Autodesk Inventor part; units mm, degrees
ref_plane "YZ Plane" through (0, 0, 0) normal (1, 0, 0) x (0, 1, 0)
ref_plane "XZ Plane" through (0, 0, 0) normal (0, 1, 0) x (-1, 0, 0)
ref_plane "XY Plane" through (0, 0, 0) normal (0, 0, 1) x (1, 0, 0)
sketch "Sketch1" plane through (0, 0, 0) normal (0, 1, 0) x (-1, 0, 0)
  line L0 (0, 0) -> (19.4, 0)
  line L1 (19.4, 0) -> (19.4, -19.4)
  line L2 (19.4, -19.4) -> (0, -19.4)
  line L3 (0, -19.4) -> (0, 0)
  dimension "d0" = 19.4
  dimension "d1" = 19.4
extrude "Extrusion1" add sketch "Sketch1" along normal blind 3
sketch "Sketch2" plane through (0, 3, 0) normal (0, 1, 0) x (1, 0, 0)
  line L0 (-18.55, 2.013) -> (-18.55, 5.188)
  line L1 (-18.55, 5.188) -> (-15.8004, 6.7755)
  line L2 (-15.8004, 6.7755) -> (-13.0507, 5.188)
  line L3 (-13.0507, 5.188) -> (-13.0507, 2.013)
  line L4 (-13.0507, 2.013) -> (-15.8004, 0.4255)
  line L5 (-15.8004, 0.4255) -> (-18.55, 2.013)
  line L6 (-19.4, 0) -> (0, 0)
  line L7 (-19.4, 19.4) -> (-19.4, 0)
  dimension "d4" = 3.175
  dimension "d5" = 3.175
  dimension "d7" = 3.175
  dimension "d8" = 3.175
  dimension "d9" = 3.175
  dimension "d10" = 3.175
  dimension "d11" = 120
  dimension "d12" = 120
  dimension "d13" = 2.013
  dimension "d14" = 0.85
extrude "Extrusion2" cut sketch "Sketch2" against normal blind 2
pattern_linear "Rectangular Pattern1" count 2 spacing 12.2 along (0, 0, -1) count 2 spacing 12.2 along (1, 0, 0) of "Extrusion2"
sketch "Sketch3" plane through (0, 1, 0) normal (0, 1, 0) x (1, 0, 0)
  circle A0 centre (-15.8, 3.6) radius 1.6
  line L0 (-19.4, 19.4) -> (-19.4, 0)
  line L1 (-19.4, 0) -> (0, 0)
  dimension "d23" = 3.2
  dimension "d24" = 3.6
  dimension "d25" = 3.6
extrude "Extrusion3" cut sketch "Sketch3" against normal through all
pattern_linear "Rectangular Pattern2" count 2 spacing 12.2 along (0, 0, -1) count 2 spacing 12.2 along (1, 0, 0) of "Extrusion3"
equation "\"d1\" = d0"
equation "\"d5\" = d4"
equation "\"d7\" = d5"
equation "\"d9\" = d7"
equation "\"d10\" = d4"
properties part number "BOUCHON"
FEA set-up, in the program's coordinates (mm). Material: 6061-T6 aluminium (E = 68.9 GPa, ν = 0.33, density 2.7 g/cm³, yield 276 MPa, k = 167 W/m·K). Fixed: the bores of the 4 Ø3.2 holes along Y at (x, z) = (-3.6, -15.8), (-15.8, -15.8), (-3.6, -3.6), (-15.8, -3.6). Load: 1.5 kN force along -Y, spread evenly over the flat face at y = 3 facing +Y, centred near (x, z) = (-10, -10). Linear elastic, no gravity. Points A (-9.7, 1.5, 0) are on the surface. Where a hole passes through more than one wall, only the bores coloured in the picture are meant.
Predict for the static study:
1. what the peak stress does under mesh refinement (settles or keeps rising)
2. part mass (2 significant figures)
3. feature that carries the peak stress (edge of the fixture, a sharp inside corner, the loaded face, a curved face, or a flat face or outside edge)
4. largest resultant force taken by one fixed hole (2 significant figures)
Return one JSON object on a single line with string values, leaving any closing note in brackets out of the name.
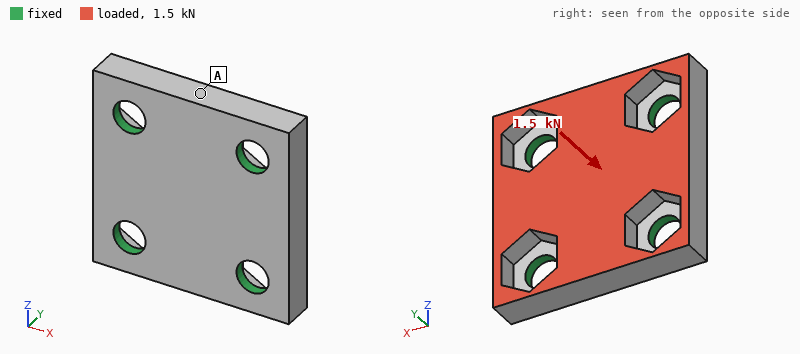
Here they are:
{"what the peak stress does under mesh refinement": "keeps rising", "part mass": "2.4 g", "feature that carries the peak stress": "edge of the fixture", "largest resultant force taken by one fixed hole": "400 N"}
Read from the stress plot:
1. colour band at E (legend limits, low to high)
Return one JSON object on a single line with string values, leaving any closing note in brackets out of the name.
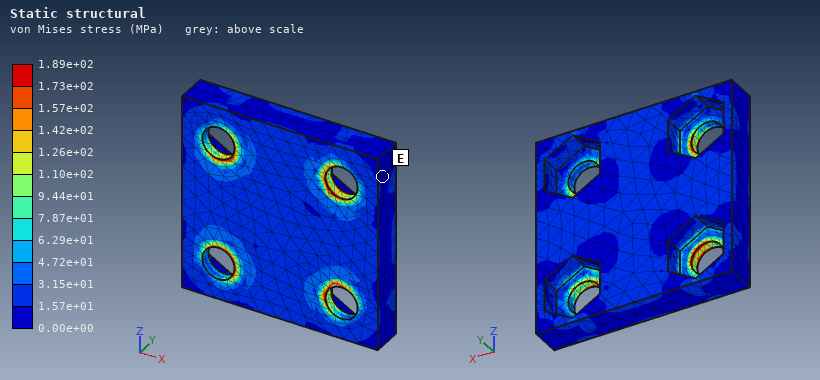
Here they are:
{"colour band at E": "0.00e+00 to 1.57e+01 MPa"}
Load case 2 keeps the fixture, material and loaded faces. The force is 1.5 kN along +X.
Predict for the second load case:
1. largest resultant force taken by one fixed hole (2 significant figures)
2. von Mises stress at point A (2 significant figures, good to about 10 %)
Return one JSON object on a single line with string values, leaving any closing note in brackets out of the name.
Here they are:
{"largest resultant force taken by one fixed hole": "410 N", "von Mises stress at point A": "15 MPa"}
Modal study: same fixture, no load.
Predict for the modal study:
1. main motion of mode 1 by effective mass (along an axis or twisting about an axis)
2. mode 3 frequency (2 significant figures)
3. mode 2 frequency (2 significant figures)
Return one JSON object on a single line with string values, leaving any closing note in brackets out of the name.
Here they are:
{"main motion of mode 1 by effective mass": "along Y", "mode 3 frequency": "59 kHz", "mode 2 frequency": "59 kHz"}
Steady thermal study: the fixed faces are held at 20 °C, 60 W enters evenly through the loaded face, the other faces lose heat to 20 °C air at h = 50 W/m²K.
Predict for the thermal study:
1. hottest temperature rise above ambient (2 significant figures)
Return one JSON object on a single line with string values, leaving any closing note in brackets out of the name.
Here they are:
{"hottest temperature rise above ambient": "21 K"}
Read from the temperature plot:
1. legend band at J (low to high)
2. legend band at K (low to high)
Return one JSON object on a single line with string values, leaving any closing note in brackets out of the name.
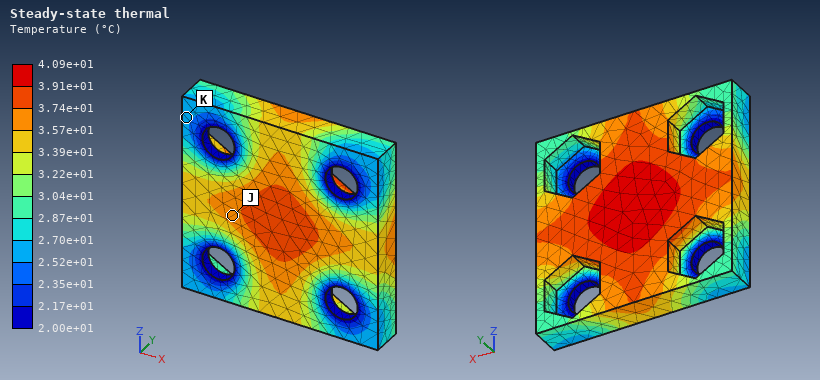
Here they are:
{"legend band at J": "3.57e+01 to 3.74e+01 °C", "legend band at K": "2.52e+01 to 2.70e+01 °C"}
